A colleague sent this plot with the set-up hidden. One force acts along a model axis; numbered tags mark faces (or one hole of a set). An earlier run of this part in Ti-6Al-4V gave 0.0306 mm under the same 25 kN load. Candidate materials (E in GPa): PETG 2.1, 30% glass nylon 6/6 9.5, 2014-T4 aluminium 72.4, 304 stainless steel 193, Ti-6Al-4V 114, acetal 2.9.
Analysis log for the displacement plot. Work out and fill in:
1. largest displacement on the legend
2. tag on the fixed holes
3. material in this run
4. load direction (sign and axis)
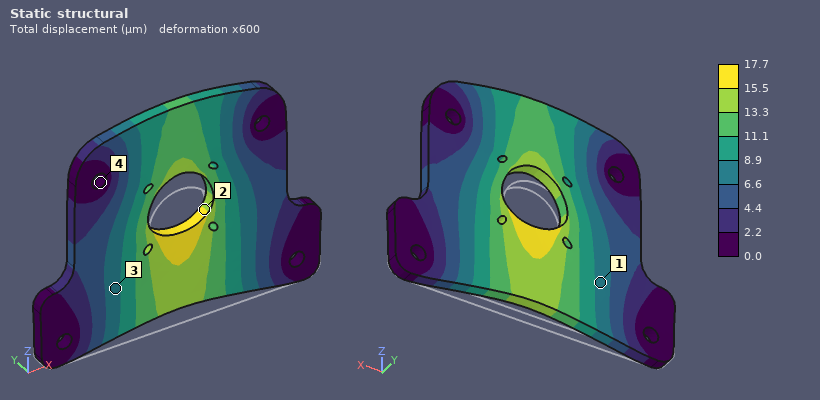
17.7 µm
4
304 stainless steel
+Z
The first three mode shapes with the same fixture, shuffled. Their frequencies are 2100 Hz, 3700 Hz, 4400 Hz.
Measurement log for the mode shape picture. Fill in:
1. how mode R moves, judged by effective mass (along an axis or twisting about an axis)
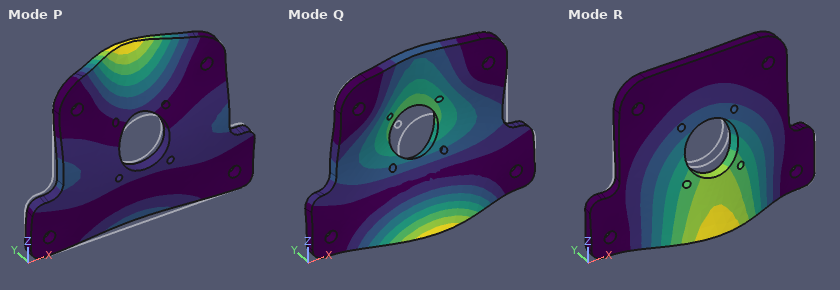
along Y
